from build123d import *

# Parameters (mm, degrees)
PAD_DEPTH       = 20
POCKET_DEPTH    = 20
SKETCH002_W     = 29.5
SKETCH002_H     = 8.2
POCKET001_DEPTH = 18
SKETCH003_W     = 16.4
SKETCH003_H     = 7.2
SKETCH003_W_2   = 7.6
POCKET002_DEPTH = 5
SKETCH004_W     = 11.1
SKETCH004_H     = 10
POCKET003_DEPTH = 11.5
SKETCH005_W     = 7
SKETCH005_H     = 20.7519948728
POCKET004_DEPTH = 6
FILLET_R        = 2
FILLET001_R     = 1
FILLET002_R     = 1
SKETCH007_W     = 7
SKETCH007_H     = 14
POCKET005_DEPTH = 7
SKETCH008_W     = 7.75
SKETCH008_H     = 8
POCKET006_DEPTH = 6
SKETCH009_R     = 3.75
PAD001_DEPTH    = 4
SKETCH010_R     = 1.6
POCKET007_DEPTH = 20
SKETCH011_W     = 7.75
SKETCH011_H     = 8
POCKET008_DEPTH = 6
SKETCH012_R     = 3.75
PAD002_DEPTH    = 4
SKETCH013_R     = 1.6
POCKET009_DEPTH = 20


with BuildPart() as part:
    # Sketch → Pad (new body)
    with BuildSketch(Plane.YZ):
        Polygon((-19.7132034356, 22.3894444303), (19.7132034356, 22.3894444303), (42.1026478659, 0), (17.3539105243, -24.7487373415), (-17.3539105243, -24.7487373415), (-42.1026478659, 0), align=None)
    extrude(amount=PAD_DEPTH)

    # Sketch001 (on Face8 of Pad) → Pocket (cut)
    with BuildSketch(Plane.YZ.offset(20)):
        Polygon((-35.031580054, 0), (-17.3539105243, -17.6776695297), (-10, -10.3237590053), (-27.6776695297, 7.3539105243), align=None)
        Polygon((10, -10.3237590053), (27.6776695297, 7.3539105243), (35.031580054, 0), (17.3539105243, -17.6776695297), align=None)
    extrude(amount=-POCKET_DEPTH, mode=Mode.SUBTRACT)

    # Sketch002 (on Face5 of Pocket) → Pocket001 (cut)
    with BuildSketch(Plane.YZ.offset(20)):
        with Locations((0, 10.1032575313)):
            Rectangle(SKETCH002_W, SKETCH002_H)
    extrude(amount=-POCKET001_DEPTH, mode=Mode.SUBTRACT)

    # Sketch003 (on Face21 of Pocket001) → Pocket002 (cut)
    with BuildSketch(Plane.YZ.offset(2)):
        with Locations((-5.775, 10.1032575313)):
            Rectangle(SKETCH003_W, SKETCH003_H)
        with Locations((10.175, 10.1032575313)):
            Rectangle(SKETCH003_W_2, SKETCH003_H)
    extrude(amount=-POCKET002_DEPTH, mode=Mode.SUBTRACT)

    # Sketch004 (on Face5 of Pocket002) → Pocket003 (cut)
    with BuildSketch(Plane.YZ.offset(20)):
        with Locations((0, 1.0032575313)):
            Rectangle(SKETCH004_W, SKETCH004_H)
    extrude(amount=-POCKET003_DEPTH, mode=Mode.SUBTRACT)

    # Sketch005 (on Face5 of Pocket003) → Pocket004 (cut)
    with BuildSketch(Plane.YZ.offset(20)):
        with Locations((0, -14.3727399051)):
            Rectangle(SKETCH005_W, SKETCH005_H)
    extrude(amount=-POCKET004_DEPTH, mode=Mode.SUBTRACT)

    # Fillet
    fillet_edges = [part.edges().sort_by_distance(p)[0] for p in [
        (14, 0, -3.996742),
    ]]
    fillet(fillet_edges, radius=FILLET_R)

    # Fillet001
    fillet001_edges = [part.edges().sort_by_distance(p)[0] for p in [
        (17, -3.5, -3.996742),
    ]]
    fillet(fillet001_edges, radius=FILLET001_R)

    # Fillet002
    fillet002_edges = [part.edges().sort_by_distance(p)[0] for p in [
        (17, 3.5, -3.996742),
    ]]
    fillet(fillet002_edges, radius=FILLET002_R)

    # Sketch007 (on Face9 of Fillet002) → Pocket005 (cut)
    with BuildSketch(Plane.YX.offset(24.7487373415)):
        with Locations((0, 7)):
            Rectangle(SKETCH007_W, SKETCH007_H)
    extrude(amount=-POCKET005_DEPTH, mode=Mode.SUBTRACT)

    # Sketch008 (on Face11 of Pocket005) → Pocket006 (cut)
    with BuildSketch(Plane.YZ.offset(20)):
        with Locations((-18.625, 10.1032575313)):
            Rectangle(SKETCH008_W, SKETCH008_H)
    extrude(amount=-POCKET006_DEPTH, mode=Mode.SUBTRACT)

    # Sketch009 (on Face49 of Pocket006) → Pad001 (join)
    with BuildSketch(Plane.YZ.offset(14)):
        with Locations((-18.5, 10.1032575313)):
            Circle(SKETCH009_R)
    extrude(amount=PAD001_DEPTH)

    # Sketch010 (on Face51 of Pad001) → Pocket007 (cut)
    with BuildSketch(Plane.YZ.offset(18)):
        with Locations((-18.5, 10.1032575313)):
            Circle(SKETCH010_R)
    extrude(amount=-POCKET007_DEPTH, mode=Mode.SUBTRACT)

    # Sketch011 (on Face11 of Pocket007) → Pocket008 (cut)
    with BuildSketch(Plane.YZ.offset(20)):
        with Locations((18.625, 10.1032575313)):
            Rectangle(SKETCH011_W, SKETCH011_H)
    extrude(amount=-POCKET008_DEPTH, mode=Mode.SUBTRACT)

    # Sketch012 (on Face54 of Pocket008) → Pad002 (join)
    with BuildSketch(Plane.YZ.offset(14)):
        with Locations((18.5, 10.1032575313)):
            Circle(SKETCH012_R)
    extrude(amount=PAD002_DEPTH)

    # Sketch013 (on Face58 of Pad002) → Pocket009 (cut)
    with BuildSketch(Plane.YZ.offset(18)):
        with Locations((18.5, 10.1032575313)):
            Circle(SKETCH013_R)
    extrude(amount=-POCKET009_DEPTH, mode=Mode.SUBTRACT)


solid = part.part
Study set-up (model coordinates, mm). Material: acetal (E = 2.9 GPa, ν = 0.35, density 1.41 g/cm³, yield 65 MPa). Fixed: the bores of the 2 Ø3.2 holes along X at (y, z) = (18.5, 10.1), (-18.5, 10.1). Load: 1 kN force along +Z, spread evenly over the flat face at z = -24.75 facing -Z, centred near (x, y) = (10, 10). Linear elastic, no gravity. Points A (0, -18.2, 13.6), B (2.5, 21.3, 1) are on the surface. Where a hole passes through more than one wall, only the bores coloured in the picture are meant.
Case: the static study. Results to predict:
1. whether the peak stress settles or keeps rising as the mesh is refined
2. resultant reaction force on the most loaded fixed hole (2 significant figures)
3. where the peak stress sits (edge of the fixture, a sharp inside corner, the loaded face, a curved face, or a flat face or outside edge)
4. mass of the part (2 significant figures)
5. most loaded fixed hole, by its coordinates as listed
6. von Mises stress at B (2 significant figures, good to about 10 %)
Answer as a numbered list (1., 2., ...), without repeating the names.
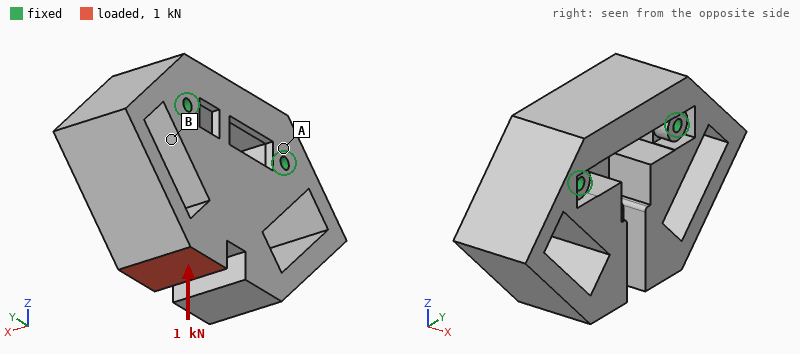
1. keeps rising
2. 820 N
3. a sharp inside corner
4. 54 g
5. (18.5, 10.1)
6. 2.3 MPa
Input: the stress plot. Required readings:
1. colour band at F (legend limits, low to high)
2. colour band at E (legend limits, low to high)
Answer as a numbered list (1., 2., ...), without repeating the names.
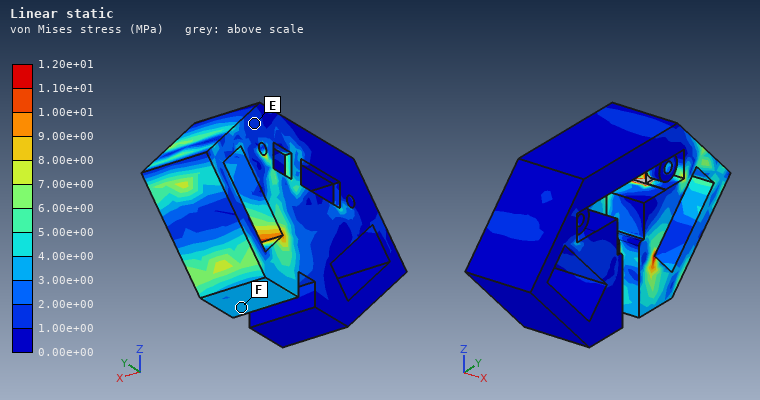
1. 3.00e+00 to 4.00e+00 MPa
2. 1.00e+00 to 2.00e+00 MPa
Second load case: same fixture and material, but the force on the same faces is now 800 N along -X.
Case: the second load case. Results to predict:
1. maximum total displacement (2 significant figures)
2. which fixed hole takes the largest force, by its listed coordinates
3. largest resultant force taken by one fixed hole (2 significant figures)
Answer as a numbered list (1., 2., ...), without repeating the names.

1. 1.0 mm
2. (18.5, 10.1)
3. 610 N
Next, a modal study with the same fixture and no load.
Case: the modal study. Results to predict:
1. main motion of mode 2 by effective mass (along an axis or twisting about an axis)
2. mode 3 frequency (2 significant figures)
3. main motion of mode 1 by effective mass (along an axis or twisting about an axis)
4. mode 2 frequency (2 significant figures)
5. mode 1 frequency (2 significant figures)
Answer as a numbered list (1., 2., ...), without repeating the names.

1. along Y
2. 2900 Hz
3. along X
4. 2700 Hz
5. 1500 Hz
